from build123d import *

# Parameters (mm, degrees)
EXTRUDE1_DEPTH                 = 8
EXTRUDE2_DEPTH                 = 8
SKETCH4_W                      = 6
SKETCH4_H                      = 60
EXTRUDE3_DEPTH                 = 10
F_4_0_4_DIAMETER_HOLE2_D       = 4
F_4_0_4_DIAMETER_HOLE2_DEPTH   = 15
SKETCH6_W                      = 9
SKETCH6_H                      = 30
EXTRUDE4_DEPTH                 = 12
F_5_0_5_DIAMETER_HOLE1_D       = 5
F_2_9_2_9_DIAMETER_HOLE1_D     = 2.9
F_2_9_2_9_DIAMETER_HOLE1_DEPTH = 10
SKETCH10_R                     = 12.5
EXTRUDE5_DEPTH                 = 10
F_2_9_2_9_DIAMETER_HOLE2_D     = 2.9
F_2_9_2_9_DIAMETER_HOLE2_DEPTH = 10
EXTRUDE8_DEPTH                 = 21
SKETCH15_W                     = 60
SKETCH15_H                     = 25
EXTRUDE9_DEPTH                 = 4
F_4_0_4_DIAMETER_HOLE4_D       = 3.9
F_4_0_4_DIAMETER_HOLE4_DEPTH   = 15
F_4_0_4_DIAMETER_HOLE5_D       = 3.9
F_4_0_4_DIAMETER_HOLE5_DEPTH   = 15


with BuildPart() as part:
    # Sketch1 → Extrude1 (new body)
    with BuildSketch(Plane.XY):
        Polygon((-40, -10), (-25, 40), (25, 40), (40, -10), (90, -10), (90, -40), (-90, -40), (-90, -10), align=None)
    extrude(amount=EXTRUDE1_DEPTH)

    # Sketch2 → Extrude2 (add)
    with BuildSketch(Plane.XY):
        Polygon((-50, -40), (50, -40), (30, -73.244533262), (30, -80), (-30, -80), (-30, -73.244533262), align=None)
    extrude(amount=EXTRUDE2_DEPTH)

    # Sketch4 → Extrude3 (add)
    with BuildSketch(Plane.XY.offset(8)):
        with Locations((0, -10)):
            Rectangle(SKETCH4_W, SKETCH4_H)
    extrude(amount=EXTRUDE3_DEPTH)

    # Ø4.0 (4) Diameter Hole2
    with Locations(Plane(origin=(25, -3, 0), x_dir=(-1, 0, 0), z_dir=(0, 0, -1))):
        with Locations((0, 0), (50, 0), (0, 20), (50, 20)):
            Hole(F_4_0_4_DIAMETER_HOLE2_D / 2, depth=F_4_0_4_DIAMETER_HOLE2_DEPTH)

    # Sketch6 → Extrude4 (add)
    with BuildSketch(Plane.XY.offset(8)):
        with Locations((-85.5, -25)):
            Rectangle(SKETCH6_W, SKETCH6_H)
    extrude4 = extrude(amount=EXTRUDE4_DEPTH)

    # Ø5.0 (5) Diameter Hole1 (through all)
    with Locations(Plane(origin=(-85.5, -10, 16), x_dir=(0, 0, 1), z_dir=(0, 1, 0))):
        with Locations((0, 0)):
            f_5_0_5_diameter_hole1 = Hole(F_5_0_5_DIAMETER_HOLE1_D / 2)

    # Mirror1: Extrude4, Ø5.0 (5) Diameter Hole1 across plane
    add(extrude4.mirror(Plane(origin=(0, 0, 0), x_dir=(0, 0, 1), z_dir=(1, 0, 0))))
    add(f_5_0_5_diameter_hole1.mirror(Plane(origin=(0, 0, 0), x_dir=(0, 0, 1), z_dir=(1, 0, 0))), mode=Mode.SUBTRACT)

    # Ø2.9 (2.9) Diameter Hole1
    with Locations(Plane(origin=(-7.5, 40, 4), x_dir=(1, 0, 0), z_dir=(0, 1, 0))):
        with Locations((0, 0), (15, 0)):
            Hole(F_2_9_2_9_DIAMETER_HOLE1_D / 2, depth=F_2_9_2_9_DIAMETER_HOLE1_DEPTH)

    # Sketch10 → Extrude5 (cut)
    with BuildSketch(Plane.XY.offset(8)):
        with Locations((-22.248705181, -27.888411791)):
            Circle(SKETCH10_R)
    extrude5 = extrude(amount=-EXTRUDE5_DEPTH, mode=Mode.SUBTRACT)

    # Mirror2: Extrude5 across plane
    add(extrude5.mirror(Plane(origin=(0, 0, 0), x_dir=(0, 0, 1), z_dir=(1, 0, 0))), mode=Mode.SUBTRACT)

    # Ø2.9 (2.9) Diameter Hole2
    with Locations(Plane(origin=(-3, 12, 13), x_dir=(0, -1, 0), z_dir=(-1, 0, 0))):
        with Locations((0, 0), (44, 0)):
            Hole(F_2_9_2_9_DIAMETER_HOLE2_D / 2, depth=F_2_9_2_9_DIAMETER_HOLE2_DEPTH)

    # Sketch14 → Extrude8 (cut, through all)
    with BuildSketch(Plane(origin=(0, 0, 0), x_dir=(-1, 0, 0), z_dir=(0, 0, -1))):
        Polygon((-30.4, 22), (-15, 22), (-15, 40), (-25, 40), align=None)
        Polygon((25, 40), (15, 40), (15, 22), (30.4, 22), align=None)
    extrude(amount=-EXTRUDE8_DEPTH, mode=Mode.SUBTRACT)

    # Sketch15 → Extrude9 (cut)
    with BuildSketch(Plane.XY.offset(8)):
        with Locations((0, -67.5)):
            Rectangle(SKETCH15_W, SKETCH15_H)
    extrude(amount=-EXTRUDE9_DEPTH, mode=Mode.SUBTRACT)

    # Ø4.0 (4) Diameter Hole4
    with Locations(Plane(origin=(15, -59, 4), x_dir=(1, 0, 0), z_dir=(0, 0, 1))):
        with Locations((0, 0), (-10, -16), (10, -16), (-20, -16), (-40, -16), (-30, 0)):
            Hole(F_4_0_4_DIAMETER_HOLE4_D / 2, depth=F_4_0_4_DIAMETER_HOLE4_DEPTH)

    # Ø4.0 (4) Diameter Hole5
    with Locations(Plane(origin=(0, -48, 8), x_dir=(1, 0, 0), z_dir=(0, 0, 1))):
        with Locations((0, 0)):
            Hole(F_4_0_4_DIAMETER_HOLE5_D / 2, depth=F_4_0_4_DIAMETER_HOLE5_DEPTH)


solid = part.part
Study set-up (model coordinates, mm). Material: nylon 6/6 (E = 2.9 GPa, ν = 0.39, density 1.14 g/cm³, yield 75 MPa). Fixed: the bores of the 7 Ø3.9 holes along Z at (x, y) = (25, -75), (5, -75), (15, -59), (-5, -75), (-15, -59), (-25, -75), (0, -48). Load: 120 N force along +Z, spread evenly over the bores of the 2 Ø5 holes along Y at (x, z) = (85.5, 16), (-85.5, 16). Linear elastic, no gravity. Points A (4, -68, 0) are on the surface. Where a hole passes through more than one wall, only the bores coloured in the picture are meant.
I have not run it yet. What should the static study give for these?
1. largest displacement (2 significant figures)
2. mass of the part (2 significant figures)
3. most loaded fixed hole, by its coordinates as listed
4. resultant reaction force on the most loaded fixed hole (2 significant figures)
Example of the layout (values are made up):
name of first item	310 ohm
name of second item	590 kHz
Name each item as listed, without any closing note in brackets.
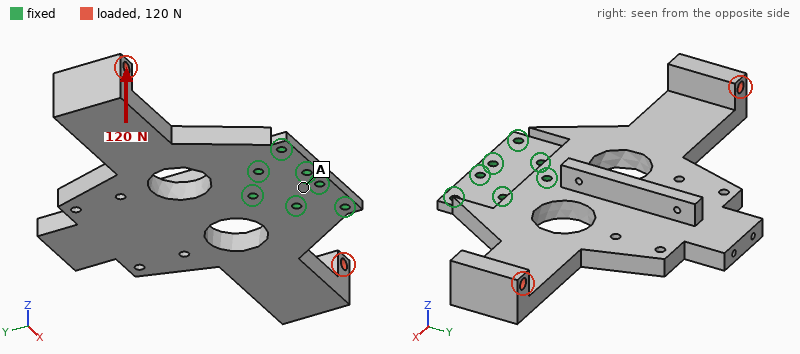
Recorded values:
largest displacement	2.6 mm
mass of the part	96 g
most loaded fixed hole, by its coordinates as listed	(0, -48)
resultant reaction force on the most loaded fixed hole	150 N
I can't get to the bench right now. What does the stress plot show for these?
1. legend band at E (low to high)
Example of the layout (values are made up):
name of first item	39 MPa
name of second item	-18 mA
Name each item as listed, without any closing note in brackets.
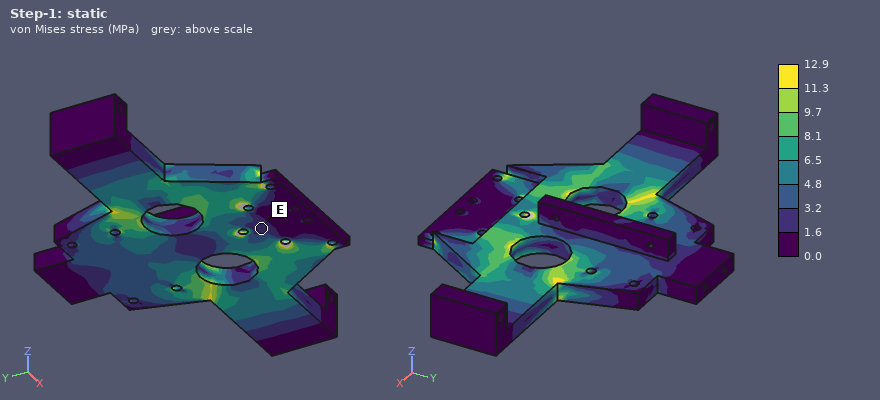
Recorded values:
legend band at E	1.6 to 3.2 MPa
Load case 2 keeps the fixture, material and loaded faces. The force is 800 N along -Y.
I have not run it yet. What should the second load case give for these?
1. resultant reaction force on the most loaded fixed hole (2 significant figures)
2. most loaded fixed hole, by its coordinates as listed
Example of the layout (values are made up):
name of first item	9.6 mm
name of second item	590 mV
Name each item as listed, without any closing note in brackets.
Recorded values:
resultant reaction force on the most loaded fixed hole	490 N
most loaded fixed hole, by its coordinates as listed	(0, -48)
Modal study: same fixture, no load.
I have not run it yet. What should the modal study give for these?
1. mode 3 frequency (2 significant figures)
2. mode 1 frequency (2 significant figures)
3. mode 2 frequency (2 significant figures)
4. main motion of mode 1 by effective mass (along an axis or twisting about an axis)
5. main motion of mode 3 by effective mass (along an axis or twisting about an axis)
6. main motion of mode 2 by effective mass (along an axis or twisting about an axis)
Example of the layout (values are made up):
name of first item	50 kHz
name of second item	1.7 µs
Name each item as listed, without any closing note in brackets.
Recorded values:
mode 3 frequency	330 Hz
mode 1 frequency	200 Hz
mode 2 frequency	240 Hz
main motion of mode 1 by effective mass	twisting about Y
main motion of mode 3 by effective mass	twisting about X
main motion of mode 2 by effective mass	along Z
